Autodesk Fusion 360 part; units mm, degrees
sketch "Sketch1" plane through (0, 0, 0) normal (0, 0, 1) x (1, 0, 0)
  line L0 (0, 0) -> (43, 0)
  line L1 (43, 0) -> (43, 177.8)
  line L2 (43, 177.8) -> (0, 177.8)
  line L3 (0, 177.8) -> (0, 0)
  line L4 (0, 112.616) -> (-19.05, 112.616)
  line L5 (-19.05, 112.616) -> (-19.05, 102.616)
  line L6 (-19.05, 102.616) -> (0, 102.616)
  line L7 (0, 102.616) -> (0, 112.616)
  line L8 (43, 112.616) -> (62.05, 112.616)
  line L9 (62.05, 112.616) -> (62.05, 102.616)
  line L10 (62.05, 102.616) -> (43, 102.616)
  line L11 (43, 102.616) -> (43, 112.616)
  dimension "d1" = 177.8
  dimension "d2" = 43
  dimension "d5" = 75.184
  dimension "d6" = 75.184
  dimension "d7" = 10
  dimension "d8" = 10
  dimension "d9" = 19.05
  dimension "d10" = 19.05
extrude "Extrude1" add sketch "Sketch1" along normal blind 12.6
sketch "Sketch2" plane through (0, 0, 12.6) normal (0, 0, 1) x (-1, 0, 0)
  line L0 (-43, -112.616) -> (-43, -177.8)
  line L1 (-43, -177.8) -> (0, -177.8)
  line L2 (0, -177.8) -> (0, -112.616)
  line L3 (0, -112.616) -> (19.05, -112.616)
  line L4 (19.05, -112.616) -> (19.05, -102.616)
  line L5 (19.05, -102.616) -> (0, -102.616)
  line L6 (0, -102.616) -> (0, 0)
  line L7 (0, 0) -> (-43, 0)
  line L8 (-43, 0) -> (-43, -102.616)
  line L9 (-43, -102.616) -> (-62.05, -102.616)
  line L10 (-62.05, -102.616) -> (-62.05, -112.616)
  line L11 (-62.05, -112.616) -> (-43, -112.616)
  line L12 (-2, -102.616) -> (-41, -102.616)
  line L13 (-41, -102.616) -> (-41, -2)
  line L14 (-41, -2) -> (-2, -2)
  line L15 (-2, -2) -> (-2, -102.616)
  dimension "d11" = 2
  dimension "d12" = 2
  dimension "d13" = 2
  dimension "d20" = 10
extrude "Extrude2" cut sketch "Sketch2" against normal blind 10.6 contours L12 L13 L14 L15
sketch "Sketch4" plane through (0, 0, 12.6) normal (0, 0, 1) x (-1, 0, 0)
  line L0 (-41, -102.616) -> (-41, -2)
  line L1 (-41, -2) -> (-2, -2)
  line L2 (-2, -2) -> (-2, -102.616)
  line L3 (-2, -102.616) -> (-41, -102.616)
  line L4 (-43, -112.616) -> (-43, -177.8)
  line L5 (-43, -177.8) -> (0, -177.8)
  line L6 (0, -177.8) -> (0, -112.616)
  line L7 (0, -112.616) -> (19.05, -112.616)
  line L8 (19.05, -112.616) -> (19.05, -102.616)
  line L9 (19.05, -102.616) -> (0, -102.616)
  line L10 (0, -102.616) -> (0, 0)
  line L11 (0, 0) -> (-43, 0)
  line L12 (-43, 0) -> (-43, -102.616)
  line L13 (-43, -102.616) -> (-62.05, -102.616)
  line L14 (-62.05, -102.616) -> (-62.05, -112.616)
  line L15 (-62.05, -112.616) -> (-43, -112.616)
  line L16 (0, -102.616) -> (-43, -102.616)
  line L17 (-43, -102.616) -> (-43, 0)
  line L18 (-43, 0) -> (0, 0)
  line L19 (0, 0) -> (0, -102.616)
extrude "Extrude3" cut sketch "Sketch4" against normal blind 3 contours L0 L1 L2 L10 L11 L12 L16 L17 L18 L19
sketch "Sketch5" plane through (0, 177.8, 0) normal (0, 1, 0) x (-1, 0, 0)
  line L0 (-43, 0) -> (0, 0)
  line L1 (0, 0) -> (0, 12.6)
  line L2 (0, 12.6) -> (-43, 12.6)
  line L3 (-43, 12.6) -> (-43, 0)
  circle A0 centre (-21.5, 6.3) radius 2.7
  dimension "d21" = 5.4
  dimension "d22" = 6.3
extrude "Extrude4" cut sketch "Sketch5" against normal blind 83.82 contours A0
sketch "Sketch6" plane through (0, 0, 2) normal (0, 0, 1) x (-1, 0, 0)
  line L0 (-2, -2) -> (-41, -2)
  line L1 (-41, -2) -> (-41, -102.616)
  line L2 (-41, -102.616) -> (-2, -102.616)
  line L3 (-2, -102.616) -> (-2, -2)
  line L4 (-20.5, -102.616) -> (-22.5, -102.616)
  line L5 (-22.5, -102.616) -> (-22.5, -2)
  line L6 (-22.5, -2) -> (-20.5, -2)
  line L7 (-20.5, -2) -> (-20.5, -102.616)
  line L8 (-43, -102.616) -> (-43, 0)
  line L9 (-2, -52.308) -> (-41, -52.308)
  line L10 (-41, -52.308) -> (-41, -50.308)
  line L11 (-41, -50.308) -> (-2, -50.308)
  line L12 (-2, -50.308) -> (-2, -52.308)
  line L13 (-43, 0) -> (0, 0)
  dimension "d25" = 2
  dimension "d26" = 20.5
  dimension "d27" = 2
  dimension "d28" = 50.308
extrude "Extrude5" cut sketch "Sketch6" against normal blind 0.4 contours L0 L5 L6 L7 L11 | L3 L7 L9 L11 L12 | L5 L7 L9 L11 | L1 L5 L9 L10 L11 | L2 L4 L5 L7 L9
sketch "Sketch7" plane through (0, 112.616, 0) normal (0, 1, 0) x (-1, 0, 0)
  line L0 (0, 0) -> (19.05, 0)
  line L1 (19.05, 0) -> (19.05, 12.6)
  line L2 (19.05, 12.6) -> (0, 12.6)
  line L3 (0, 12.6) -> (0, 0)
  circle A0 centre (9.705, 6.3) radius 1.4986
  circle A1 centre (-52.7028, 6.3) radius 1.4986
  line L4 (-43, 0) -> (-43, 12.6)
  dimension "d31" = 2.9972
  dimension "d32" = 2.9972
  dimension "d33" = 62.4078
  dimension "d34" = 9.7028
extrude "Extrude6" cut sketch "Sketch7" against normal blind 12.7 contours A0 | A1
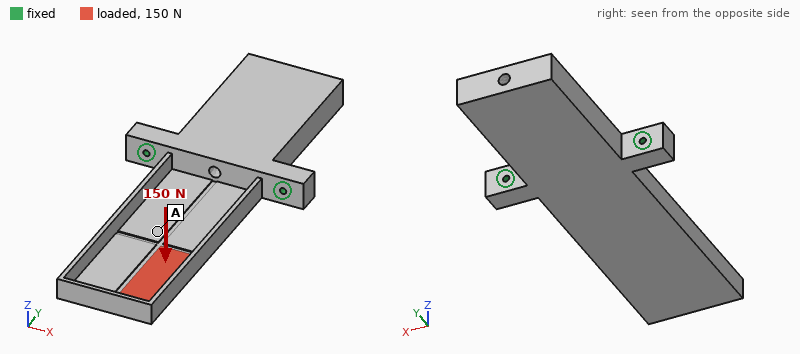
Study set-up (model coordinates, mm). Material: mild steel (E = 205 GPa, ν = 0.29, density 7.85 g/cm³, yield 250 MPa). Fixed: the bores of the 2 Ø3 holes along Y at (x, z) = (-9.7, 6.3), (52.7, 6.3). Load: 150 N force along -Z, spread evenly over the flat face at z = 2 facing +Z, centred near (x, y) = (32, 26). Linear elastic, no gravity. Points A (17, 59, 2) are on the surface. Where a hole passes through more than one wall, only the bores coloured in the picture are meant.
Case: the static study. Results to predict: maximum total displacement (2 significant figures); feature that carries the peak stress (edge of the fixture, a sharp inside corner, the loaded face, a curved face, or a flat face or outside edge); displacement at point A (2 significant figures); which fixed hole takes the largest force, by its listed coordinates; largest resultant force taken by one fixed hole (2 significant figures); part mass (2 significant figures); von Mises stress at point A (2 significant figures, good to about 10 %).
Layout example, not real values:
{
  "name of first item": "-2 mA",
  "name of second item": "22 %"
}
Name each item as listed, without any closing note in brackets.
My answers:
{
  "maximum total displacement": "0.40 mm",
  "feature that carries the peak stress": "a flat face or outside edge",
  "displacement at point A": "0.093 mm",
  "which fixed hole takes the largest force, by its listed coordinates": "(52.7, 6.3)",
  "largest resultant force taken by one fixed hole": "130 N",
  "part mass": "440 g",
  "von Mises stress at point A": "18 MPa"
}
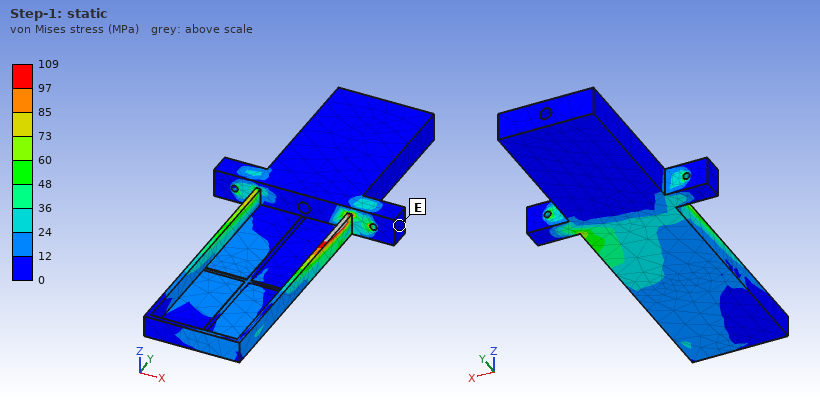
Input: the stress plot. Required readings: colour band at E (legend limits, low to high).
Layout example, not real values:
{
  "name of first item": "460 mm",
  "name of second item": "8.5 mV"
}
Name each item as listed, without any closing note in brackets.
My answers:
{
  "colour band at E": "0 to 12 MPa"
}
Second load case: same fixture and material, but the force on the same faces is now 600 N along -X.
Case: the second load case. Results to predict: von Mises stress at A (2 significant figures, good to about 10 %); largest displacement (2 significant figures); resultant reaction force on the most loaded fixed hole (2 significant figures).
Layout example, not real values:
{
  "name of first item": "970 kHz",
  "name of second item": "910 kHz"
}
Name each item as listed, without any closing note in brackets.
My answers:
{
  "von Mises stress at A": "32 MPa",
  "largest displacement": "0.16 mm",
  "resultant reaction force on the most loaded fixed hole": "980 N"
}
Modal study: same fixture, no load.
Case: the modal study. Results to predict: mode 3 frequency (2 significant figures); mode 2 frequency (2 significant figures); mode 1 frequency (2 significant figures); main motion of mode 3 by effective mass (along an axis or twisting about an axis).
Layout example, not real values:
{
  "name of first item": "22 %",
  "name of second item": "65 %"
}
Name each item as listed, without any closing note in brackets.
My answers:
{
  "mode 3 frequency": "1100 Hz",
  "mode 2 frequency": "960 Hz",
  "mode 1 frequency": "520 Hz",
  "main motion of mode 3 by effective mass": "along Z"
}
